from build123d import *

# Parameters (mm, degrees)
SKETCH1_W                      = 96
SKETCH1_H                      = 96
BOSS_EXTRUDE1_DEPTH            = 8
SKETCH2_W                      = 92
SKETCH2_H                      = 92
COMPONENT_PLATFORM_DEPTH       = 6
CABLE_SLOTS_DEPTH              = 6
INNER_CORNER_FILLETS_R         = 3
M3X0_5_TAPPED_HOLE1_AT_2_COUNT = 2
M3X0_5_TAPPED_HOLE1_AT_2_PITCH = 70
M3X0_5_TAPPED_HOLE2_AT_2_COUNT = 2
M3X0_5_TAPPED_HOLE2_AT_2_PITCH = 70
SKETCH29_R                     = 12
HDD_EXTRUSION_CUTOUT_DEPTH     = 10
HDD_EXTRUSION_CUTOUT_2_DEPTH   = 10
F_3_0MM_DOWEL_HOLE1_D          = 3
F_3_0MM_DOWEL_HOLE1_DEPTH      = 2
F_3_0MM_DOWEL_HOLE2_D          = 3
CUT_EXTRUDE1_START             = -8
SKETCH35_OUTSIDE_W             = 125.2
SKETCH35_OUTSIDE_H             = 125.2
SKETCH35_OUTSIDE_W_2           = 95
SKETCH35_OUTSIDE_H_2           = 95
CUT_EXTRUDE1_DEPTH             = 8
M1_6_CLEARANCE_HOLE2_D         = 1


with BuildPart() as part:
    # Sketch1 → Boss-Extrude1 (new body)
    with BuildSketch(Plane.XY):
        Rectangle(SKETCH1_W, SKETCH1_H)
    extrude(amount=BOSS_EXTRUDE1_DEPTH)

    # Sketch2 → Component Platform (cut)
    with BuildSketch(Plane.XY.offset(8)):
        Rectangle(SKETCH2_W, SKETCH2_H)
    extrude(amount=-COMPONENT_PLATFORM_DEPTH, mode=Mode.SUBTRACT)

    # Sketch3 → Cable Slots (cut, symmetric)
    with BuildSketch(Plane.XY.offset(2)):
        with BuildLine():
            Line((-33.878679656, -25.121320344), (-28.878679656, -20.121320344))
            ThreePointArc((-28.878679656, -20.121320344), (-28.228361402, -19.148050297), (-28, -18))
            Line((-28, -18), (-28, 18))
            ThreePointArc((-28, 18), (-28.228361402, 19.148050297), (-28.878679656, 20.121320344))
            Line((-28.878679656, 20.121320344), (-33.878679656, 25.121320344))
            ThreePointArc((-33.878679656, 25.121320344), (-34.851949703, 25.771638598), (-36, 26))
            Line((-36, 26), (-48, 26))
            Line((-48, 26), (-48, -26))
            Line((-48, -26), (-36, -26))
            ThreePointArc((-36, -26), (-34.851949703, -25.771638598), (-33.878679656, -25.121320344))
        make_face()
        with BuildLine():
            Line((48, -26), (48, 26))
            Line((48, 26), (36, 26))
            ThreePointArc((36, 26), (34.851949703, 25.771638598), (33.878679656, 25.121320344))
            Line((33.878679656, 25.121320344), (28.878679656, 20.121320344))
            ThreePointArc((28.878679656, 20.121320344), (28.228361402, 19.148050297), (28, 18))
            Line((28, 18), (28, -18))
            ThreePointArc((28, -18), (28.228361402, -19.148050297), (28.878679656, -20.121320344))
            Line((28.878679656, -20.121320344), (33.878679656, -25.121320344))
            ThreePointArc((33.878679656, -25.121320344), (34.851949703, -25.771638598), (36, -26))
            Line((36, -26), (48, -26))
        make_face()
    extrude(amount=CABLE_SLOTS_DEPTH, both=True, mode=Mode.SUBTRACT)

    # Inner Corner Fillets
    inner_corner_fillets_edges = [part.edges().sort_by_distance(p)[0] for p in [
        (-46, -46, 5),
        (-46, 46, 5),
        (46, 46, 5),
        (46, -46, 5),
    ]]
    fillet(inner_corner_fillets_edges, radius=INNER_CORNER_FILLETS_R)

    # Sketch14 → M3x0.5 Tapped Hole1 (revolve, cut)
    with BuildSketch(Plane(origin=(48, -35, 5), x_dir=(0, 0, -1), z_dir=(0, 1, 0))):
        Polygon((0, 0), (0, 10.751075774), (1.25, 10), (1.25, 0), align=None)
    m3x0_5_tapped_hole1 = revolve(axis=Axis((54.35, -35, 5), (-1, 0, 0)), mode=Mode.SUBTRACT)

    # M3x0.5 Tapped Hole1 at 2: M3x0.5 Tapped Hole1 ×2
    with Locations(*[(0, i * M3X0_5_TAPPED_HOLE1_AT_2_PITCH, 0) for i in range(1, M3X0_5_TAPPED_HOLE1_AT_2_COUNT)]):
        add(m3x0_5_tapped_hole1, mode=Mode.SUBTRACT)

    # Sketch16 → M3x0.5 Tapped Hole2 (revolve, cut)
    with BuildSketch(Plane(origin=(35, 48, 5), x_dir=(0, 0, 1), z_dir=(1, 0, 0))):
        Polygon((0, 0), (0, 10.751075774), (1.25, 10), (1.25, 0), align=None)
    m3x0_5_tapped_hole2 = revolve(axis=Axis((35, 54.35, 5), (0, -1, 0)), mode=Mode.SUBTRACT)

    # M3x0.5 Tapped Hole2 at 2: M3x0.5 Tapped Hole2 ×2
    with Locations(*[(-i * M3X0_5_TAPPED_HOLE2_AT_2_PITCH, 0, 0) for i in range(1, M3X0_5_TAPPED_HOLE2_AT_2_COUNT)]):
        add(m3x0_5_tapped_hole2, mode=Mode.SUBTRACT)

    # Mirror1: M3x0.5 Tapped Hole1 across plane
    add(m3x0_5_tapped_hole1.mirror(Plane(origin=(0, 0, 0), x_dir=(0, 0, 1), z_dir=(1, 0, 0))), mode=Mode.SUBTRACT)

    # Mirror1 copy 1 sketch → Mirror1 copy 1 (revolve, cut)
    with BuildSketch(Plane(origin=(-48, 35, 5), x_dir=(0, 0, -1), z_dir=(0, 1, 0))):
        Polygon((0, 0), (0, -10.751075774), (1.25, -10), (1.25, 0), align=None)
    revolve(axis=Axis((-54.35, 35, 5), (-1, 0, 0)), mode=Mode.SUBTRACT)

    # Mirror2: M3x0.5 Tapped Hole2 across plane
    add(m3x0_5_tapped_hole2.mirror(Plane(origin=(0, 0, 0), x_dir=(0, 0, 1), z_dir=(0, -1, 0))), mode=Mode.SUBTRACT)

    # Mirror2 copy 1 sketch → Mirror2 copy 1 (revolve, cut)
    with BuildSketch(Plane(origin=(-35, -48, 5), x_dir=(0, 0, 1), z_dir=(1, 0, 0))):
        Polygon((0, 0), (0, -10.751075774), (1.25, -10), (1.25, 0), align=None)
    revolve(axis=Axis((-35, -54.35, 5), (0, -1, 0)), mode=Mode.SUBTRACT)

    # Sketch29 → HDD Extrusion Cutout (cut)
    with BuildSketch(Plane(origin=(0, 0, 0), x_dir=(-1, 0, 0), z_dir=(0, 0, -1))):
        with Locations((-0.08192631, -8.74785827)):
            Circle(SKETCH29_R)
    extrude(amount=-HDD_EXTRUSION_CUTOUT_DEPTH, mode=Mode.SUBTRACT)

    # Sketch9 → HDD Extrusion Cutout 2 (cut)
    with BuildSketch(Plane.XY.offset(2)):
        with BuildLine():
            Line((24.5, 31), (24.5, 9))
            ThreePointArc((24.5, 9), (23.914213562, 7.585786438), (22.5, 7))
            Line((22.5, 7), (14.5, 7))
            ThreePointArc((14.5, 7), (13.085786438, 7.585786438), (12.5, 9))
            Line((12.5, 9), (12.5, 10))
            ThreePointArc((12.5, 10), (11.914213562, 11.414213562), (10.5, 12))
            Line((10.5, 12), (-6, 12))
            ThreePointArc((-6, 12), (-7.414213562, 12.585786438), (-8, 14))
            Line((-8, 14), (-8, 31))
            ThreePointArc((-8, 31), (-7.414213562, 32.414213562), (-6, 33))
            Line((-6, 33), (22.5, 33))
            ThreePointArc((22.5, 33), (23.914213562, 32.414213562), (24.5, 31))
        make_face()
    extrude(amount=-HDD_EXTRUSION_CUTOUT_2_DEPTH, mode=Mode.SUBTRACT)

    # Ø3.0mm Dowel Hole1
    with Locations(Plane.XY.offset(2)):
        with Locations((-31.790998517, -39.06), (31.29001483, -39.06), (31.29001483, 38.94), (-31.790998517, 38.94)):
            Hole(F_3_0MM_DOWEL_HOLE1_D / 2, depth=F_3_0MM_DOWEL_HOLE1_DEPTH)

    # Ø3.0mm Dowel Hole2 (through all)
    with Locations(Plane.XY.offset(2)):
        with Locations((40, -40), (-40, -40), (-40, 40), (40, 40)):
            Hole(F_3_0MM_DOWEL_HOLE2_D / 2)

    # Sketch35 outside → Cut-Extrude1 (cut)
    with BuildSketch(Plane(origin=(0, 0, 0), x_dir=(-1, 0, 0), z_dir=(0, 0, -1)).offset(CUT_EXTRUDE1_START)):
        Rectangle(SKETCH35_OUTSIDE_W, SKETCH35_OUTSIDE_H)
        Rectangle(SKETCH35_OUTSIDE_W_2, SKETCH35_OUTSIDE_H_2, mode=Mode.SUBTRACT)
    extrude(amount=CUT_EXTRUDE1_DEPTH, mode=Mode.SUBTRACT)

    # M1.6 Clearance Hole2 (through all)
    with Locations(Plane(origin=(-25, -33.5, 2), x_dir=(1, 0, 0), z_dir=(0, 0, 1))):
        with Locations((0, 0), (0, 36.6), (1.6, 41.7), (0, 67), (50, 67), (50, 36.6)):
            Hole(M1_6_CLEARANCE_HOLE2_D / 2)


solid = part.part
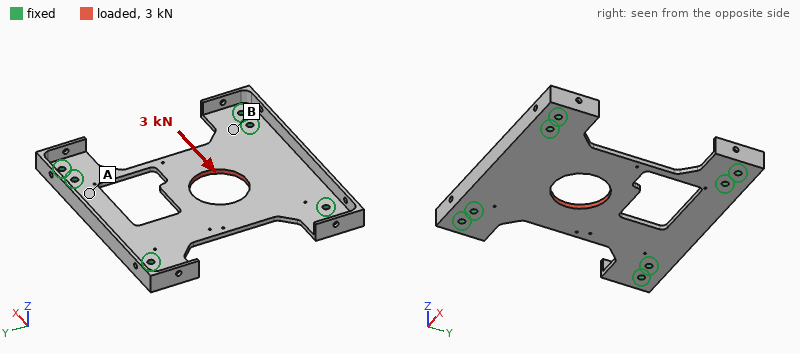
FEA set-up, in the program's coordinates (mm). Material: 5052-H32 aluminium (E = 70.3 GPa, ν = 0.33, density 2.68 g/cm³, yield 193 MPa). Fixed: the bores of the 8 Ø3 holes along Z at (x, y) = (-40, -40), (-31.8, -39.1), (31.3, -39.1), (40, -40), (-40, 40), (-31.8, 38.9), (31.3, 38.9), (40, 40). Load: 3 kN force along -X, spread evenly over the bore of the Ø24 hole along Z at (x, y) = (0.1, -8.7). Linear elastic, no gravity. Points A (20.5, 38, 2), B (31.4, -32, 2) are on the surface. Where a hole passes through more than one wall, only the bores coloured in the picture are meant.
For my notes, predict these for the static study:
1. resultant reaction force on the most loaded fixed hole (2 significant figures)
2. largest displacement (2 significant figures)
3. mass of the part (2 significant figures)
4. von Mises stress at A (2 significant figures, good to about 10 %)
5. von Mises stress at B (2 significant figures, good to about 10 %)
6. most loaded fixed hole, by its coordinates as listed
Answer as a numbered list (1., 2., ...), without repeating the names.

1. 950 N
2. 43 µm
3. 38 g
4. 8.5 MPa
5. 27 MPa
6. (-31.8, -39.1)
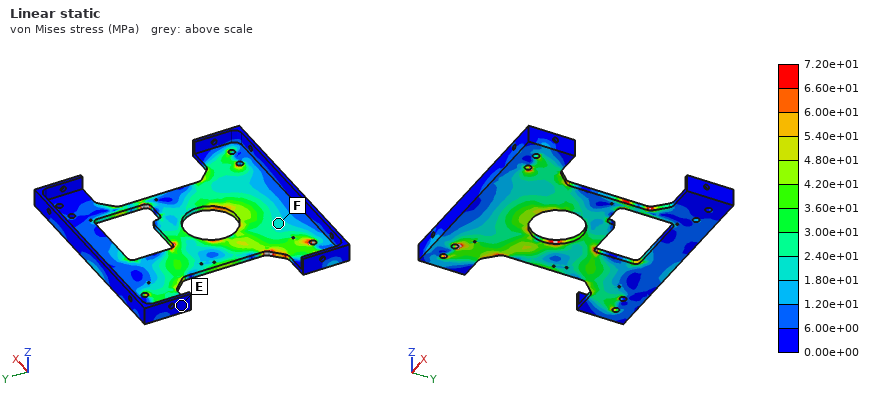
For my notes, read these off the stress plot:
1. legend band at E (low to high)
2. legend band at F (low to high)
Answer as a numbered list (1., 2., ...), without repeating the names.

1. 0.00e+00 to 6.00e+00 MPa
2. 1.80e+01 to 2.40e+01 MPa
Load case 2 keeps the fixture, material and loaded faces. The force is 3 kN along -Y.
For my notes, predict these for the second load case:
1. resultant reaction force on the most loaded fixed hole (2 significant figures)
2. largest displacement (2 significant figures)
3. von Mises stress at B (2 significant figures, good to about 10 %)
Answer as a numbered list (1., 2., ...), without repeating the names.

1. 1.1 kN
2. 33 µm
3. 34 MPa
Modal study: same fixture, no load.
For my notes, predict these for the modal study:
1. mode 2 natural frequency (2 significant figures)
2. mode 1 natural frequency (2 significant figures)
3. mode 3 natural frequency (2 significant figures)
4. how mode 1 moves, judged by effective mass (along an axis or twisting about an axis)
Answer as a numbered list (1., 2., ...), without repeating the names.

1. 2400 Hz
2. 1400 Hz
3. 3300 Hz
4. along Z
